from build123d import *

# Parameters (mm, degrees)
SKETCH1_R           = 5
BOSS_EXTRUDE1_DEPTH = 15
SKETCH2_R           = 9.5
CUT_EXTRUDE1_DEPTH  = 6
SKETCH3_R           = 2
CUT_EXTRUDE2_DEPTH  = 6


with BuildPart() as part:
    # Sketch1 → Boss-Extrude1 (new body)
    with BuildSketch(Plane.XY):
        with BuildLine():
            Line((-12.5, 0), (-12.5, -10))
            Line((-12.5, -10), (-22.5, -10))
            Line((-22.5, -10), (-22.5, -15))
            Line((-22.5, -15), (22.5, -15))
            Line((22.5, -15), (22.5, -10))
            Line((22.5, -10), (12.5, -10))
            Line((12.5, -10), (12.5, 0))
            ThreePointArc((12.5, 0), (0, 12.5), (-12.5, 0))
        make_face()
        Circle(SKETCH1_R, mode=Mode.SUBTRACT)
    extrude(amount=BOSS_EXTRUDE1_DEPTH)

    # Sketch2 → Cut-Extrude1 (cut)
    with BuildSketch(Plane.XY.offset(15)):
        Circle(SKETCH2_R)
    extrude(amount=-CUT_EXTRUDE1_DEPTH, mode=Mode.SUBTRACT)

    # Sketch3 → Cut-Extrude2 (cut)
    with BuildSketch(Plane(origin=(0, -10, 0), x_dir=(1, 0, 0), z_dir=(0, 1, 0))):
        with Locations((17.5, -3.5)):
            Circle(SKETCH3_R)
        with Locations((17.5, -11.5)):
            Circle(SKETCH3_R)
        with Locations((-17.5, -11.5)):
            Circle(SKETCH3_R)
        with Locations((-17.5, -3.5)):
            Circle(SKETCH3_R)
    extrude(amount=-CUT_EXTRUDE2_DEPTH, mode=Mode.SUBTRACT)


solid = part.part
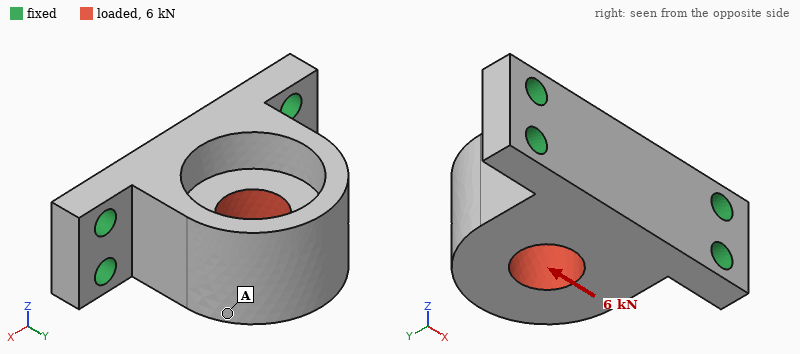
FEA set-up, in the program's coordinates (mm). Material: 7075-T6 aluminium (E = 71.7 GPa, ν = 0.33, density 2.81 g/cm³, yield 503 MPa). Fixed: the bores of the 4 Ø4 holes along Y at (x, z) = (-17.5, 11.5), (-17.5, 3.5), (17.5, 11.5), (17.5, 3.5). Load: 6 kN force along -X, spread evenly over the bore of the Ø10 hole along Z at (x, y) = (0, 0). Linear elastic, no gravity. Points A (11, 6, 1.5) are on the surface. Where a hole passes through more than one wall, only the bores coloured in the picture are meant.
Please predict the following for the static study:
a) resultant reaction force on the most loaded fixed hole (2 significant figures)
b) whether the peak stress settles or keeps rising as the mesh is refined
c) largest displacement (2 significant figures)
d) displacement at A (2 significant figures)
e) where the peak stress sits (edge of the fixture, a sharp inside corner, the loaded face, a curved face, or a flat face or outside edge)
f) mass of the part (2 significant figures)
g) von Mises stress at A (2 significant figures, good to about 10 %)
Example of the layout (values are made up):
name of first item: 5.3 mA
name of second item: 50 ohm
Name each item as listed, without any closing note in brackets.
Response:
resultant reaction force on the most loaded fixed hole: 2.2 kN
whether the peak stress settles or keeps rising as the mesh is refined: keeps rising
largest displacement: 51 µm
displacement at A: 45 µm
where the peak stress sits: edge of the fixture
mass of the part: 23 g
von Mises stress at A: 31 MPa
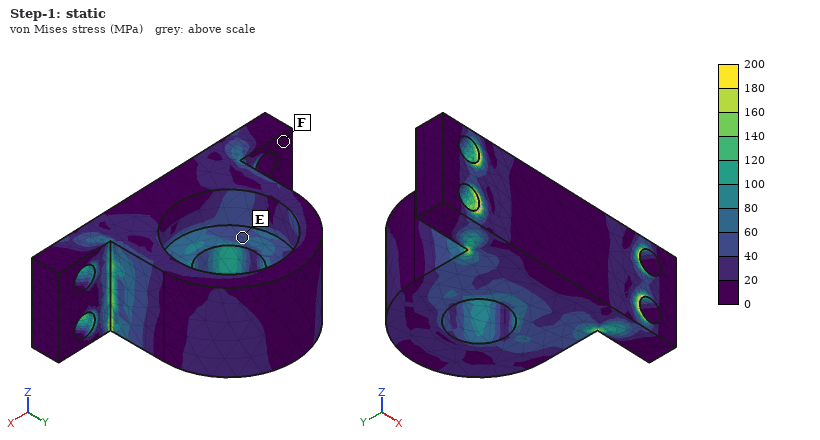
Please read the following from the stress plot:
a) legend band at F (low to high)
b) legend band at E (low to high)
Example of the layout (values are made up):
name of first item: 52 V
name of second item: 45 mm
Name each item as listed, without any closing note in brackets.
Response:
legend band at F: 0 to 20 MPa
legend band at E: 40 to 60 MPa
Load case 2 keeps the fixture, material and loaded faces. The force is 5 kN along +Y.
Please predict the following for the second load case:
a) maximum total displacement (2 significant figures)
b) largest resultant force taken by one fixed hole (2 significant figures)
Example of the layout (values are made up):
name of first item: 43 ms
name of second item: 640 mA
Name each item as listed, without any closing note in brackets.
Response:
maximum total displacement: 53 µm
largest resultant force taken by one fixed hole: 2.1 kN
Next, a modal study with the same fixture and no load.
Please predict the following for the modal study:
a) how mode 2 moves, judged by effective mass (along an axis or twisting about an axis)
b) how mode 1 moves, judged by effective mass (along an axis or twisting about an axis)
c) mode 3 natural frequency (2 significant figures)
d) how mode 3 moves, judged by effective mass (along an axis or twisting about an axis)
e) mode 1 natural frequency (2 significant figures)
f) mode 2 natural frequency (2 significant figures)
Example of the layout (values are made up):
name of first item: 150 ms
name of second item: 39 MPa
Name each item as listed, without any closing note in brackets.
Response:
how mode 2 moves, judged by effective mass: along X
how mode 1 moves, judged by effective mass: along Z
mode 3 natural frequency: 20 kHz
how mode 3 moves, judged by effective mass: along Y
mode 1 natural frequency: 7900 Hz
mode 2 natural frequency: 16 kHz
